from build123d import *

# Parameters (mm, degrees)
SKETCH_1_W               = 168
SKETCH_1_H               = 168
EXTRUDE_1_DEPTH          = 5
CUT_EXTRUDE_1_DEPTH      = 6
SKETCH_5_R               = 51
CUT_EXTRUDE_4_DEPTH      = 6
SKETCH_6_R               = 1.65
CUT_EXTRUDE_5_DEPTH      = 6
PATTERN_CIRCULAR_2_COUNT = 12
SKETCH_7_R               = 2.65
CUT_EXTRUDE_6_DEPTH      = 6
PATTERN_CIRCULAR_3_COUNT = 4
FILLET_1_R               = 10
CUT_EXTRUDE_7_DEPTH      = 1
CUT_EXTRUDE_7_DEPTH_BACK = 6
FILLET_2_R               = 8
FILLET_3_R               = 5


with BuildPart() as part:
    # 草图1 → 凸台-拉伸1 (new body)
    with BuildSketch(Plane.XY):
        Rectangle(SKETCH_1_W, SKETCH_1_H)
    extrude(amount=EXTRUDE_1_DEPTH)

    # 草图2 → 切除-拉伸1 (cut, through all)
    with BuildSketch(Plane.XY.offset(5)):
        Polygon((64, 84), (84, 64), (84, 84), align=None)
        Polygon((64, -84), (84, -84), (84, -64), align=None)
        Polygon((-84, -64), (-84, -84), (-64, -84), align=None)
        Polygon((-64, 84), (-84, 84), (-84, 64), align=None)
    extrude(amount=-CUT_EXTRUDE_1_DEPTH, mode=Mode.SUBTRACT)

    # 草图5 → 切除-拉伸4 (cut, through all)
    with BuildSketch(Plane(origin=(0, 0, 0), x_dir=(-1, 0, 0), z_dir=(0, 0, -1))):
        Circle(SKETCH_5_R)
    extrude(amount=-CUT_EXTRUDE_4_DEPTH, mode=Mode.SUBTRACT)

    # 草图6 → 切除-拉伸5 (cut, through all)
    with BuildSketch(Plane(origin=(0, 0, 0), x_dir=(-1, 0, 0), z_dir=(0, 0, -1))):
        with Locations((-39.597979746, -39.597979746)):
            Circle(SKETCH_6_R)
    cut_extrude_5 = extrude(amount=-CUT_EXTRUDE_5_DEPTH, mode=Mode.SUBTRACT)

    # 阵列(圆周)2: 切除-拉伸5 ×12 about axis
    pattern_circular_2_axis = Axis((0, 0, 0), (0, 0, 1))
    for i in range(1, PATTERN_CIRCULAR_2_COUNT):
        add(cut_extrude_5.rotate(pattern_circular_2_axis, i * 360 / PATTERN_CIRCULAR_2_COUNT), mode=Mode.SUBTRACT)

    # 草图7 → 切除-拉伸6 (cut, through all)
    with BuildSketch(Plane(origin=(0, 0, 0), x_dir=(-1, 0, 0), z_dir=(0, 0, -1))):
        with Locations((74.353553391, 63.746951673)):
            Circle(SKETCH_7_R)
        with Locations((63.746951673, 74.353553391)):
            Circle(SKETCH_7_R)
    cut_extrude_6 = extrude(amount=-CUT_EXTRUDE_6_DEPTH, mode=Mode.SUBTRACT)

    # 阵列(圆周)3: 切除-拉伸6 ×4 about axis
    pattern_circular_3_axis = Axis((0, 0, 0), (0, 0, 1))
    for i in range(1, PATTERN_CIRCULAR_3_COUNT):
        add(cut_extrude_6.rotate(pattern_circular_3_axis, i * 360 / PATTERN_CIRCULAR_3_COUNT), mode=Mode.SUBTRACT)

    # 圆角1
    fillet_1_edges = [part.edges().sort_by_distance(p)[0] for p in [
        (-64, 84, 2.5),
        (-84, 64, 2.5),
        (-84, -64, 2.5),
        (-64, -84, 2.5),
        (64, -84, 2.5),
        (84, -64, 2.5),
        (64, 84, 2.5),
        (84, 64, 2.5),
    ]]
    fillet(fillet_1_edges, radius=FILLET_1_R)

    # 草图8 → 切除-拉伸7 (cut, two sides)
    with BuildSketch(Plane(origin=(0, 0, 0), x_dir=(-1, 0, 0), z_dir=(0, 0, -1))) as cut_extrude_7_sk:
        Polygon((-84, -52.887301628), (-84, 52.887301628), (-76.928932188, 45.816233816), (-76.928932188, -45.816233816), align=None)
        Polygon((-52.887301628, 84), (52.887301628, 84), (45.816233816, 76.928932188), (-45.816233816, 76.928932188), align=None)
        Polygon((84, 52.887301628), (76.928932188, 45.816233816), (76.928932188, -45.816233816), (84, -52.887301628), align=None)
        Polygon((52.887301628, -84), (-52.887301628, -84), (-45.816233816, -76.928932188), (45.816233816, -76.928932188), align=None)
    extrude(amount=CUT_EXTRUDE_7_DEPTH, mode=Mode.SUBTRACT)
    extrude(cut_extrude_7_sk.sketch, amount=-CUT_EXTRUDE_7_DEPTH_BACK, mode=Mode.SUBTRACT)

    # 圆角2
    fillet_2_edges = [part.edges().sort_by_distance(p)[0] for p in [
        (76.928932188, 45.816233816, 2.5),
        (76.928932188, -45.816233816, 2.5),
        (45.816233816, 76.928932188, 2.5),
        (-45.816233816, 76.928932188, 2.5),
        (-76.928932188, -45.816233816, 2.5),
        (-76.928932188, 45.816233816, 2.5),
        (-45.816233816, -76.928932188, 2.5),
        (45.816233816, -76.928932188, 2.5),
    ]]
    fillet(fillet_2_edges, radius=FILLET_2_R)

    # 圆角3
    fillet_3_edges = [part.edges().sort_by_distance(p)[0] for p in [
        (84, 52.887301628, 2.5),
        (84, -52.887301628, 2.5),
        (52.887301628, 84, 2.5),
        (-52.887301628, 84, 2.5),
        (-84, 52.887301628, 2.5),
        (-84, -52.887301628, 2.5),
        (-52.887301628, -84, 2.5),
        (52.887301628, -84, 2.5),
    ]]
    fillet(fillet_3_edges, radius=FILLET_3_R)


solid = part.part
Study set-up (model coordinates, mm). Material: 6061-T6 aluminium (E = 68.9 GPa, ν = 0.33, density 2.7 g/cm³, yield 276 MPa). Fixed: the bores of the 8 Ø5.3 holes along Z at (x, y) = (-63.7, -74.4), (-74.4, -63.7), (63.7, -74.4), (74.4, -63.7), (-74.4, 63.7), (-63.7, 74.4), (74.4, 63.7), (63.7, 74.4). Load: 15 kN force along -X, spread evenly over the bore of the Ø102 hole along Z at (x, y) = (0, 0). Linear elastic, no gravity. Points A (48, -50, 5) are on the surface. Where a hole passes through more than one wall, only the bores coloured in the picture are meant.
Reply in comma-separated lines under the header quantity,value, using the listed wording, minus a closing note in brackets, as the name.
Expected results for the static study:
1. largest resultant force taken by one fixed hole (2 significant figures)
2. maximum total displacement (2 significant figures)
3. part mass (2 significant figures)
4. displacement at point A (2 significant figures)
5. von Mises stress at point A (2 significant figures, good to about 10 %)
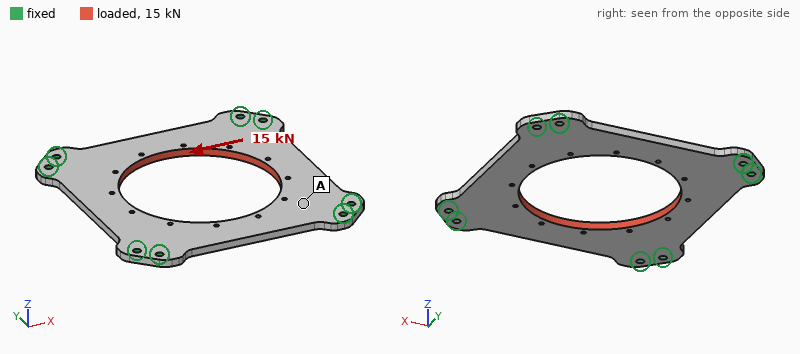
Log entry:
quantity,value
largest resultant force taken by one fixed hole,3.3 kN
maximum total displacement,52 µm
part mass,220 g
displacement at point A,18 µm
von Mises stress at point A,12 MPa
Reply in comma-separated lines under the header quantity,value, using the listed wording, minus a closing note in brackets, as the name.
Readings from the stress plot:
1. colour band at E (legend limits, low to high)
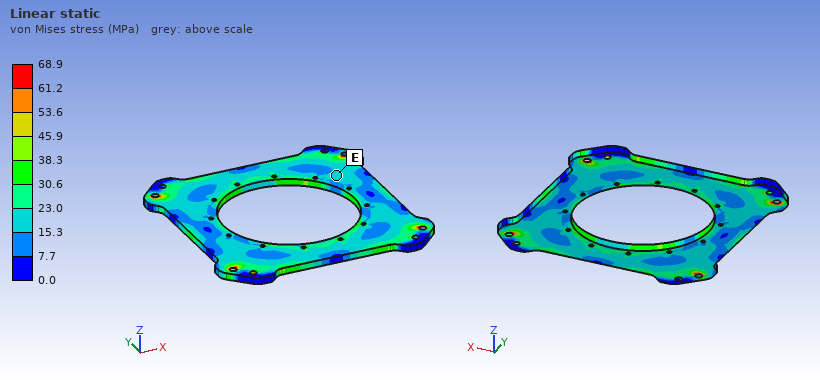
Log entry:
quantity,value
colour band at E,15.3 to 23.0 MPa
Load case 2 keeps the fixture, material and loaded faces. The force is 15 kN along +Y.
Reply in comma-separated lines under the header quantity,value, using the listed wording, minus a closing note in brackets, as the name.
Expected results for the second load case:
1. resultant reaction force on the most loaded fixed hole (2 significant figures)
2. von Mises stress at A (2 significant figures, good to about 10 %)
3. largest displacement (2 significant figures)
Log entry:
quantity,value
resultant reaction force on the most loaded fixed hole,3.3 kN
von Mises stress at A,12 MPa
largest displacement,52 µm
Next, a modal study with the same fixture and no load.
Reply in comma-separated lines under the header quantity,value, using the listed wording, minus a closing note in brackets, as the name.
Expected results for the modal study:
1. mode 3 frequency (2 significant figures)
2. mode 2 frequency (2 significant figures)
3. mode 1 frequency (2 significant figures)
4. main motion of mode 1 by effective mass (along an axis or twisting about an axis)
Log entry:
quantity,value
mode 3 frequency,1600 Hz
mode 2 frequency,1600 Hz
mode 1 frequency,1400 Hz
main motion of mode 1 by effective mass,along Z
